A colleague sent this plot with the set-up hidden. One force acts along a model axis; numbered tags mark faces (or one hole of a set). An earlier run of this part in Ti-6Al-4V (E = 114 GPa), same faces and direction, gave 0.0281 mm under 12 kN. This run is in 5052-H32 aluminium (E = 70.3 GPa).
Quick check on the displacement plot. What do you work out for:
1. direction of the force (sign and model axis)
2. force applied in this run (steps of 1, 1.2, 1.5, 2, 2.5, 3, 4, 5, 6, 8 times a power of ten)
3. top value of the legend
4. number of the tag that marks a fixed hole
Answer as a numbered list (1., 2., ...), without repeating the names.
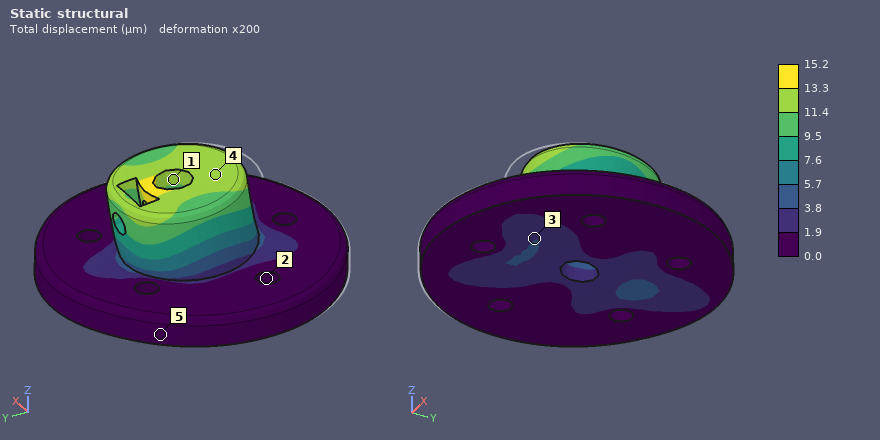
1. +Y
2. 4 kN
3. 15.2 µm
4. 2
